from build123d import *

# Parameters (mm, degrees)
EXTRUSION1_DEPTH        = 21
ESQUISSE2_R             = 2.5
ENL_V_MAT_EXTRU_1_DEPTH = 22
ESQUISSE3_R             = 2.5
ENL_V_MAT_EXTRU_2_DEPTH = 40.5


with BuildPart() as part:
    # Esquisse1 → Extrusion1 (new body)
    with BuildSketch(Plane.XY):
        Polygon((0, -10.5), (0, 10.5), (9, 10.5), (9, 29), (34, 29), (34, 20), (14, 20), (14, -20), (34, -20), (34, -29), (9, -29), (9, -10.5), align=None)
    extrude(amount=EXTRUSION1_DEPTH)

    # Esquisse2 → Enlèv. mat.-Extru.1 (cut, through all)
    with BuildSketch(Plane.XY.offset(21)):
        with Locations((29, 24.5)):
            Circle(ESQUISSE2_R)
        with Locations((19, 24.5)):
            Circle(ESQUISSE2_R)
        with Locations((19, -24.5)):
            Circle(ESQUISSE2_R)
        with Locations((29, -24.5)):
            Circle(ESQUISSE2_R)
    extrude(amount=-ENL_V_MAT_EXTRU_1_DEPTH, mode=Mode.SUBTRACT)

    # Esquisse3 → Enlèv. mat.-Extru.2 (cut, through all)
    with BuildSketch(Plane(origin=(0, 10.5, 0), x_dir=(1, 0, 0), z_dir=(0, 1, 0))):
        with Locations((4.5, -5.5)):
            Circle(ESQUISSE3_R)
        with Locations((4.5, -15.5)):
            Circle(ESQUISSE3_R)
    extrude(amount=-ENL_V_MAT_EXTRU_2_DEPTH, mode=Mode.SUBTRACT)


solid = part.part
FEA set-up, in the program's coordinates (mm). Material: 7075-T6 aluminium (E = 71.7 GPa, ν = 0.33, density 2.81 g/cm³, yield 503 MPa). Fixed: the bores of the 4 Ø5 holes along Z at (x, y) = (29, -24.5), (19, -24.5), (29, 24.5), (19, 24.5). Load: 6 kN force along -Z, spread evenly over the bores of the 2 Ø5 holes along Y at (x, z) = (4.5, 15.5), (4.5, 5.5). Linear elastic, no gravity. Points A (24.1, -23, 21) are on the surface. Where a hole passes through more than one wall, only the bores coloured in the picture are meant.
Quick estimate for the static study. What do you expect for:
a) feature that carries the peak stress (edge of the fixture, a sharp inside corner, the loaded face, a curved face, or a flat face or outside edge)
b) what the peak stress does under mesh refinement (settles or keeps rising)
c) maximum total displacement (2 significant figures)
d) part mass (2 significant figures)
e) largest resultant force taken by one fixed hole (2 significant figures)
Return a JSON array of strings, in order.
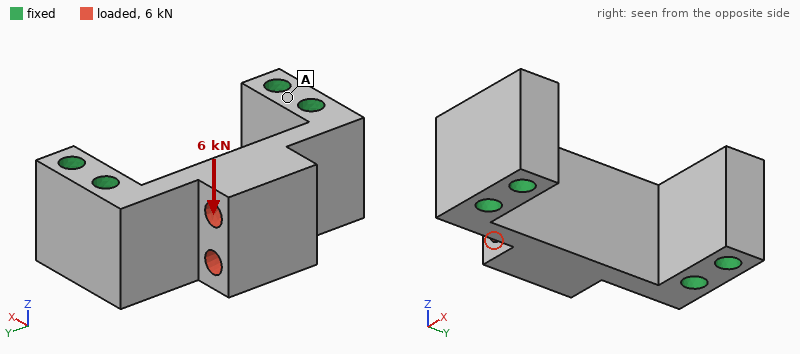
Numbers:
["a sharp inside corner", "keeps rising", "0.14 mm", "43 g", "3.0 kN"]
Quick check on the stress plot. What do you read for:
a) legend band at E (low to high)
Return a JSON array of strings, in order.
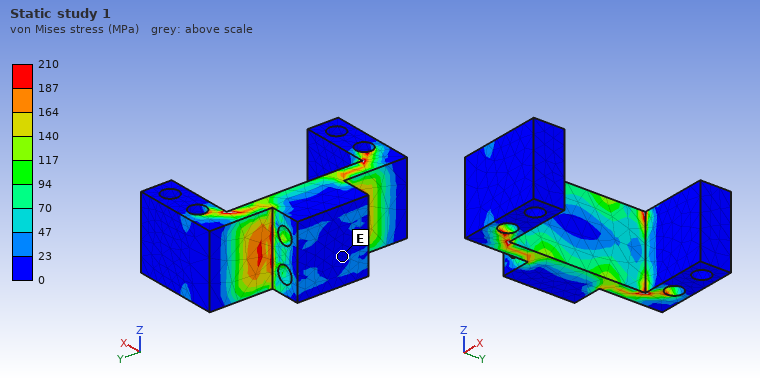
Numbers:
["0 to 23 MPa"]
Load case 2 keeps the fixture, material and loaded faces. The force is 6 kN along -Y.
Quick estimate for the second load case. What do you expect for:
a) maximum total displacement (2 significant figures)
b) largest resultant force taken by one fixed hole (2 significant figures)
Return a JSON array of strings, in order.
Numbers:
["28 µm", "3.4 kN"]
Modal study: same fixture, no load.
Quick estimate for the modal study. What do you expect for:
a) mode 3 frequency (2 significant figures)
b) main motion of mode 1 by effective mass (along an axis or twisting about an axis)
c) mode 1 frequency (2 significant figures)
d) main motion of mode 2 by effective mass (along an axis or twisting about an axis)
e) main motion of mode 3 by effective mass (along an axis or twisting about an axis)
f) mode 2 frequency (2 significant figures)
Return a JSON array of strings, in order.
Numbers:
["19 kHz", "along Z", "11 kHz", "along X", "along Z", "12 kHz"]
